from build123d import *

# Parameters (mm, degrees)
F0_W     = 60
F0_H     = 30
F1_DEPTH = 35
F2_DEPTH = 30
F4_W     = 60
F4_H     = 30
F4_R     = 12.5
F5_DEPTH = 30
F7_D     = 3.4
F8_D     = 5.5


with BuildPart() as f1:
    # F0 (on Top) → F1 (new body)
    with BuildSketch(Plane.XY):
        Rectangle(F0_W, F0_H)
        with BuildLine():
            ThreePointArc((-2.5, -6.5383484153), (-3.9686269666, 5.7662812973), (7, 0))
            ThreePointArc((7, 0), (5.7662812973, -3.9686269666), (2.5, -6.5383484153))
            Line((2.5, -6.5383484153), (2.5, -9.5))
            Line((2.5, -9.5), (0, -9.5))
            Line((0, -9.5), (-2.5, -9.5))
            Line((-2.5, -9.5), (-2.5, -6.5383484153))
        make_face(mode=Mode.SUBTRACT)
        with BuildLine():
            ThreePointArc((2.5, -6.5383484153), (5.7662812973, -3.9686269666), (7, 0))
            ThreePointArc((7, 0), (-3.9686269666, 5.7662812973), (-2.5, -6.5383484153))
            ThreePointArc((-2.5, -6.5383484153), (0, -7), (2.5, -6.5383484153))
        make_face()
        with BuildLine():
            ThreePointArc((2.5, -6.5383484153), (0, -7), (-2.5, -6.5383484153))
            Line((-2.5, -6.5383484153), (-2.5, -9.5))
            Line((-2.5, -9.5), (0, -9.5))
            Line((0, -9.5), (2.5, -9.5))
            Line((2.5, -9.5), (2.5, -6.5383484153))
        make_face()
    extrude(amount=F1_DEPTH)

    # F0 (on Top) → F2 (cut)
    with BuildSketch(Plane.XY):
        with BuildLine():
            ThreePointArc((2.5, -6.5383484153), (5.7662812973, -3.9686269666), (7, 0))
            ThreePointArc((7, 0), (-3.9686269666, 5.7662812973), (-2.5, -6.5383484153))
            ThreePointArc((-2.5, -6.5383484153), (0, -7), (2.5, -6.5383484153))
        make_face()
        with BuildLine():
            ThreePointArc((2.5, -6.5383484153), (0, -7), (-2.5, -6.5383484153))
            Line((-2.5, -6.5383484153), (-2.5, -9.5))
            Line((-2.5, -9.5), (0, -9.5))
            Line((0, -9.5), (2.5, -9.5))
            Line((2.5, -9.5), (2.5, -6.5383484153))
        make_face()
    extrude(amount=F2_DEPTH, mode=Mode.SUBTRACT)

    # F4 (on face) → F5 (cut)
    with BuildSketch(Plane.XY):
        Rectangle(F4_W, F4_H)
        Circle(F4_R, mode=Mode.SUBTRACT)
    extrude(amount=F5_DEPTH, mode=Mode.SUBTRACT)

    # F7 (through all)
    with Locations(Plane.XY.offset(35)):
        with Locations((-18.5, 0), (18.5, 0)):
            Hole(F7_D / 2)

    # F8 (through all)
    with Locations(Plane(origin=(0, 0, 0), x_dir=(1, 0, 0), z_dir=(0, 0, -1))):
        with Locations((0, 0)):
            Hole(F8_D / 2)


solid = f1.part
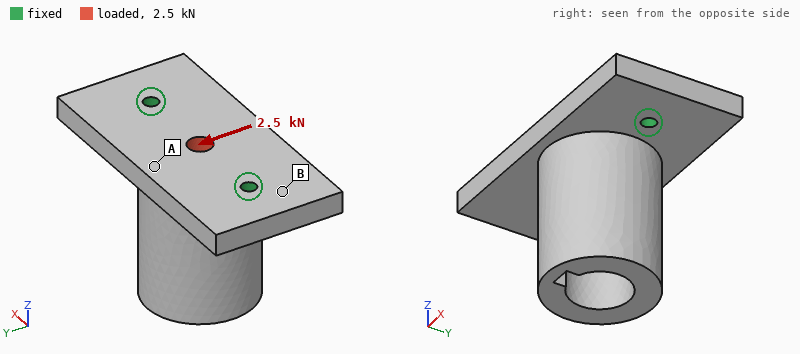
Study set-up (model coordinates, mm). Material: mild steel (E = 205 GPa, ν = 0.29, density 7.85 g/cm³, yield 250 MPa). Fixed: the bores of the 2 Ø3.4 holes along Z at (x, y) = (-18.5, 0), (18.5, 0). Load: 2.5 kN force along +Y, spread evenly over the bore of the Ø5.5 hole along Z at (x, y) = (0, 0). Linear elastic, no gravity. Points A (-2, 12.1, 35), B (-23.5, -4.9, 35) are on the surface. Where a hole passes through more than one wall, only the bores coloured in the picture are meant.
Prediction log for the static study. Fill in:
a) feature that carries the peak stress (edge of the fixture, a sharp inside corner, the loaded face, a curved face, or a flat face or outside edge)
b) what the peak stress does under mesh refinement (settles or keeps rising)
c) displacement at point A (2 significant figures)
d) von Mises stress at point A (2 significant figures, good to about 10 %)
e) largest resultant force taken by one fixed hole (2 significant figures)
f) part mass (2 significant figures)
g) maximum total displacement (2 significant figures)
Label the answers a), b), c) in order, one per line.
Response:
a) edge of the fixture
b) keeps rising
c) 2.6 µm
d) 18 MPa
e) 1.3 kN
f) 150 g
g) 3.3 µm
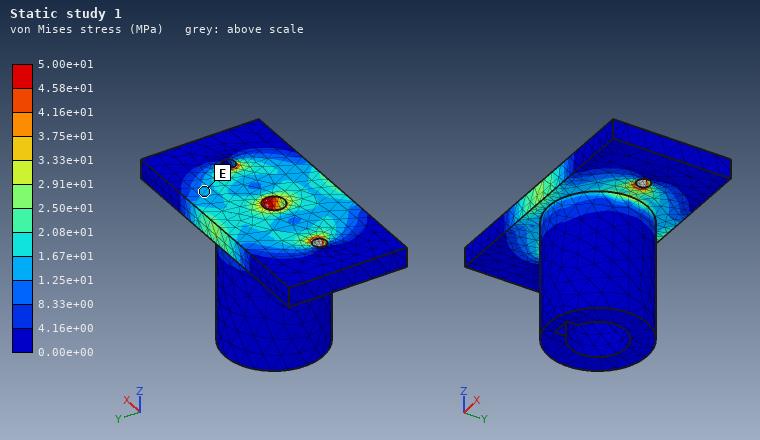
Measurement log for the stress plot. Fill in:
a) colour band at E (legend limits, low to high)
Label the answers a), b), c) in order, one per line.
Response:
a) 1.25e+01 to 1.67e+01 MPa
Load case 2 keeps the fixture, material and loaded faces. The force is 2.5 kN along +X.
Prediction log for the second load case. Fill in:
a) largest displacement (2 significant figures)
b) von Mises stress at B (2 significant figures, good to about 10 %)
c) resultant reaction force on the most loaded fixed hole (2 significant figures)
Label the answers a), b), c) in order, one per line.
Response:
a) 1.7 µm
b) 5.9 MPa
c) 1.3 kN
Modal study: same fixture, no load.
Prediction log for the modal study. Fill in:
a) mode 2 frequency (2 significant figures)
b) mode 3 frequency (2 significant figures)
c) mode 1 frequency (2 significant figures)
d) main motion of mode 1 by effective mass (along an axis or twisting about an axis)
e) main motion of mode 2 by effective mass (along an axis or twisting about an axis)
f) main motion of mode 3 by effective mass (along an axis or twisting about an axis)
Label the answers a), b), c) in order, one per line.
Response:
a) 8400 Hz
b) 11 kHz
c) 3300 Hz
d) along Y
e) along X
f) along Z
